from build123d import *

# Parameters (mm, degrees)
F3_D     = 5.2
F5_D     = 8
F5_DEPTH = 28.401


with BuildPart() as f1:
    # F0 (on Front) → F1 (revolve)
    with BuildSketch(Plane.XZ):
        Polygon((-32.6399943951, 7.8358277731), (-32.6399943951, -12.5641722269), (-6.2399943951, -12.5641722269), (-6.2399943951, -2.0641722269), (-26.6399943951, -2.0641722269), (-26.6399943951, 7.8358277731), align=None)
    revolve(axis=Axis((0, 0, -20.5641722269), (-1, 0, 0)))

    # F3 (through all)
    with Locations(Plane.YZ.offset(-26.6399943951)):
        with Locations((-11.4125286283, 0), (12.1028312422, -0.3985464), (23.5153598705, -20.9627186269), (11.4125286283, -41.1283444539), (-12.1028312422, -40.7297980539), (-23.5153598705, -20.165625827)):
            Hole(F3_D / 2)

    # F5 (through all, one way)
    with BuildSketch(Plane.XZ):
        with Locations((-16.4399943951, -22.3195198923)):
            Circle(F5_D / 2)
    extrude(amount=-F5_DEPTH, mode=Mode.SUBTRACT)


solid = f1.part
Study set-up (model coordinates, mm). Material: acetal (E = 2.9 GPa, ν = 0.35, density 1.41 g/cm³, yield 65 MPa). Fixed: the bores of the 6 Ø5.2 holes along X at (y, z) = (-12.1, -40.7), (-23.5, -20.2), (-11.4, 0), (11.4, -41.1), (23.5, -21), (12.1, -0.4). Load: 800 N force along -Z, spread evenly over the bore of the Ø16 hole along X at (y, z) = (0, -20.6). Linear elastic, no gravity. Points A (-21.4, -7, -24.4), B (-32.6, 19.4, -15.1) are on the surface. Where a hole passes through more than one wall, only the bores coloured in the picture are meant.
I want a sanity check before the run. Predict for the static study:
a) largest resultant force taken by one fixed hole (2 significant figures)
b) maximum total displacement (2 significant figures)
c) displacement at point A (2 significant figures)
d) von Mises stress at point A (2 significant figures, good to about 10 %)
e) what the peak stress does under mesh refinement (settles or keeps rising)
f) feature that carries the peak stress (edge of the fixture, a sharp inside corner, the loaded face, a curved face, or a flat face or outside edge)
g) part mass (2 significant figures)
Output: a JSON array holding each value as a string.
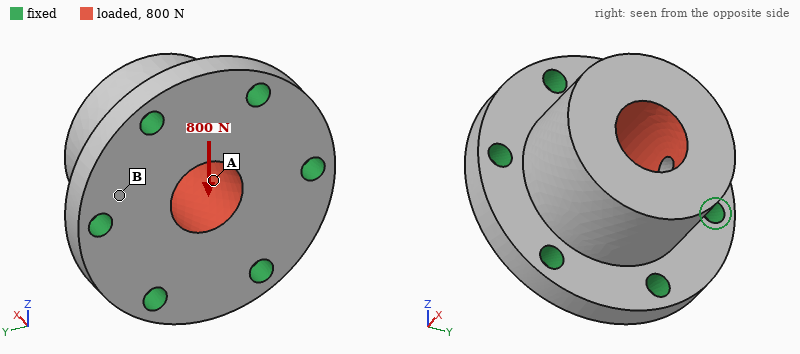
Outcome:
["210 N", "36 µm", "16 µm", "1.9 MPa", "keeps rising", "edge of the fixture", "43 g"]
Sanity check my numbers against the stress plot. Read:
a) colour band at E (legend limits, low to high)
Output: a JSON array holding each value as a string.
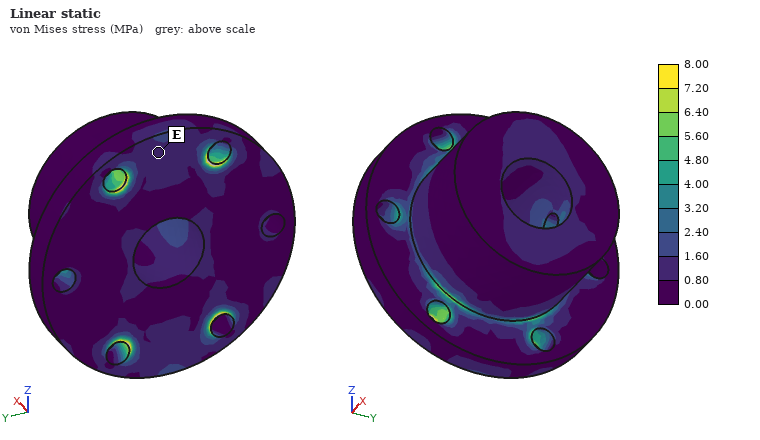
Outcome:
["0.80 to 1.60 MPa"]
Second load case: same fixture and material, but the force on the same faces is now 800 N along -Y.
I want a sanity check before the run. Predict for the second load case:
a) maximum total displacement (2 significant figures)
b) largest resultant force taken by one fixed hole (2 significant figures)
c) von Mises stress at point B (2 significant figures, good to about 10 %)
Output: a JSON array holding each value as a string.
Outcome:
["34 µm", "230 N", "0.67 MPa"]
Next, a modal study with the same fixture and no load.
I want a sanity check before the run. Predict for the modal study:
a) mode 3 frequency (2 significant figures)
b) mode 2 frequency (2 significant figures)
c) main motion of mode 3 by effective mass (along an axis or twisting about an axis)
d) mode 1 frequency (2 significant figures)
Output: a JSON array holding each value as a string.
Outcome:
["6100 Hz", "5000 Hz", "along X", "4900 Hz"]
